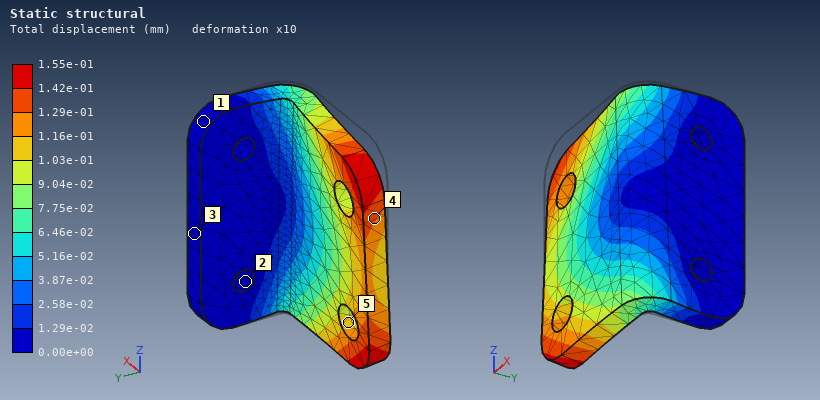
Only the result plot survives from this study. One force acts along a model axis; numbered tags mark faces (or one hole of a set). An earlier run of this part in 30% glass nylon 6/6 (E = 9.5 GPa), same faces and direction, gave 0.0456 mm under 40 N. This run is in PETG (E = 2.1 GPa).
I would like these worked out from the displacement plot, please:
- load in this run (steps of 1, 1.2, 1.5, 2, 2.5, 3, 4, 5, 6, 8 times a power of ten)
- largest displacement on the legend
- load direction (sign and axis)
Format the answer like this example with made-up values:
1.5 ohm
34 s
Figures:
30 N
1.55e-01 mm
-Z
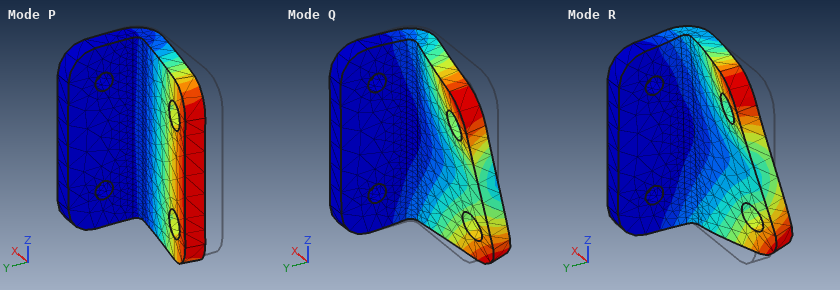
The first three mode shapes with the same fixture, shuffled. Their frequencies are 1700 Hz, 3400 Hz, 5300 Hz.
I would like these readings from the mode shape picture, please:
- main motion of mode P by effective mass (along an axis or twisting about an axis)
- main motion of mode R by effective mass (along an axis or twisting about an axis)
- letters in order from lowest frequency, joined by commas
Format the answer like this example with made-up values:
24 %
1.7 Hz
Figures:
along Y
along Z
P, Q, R
